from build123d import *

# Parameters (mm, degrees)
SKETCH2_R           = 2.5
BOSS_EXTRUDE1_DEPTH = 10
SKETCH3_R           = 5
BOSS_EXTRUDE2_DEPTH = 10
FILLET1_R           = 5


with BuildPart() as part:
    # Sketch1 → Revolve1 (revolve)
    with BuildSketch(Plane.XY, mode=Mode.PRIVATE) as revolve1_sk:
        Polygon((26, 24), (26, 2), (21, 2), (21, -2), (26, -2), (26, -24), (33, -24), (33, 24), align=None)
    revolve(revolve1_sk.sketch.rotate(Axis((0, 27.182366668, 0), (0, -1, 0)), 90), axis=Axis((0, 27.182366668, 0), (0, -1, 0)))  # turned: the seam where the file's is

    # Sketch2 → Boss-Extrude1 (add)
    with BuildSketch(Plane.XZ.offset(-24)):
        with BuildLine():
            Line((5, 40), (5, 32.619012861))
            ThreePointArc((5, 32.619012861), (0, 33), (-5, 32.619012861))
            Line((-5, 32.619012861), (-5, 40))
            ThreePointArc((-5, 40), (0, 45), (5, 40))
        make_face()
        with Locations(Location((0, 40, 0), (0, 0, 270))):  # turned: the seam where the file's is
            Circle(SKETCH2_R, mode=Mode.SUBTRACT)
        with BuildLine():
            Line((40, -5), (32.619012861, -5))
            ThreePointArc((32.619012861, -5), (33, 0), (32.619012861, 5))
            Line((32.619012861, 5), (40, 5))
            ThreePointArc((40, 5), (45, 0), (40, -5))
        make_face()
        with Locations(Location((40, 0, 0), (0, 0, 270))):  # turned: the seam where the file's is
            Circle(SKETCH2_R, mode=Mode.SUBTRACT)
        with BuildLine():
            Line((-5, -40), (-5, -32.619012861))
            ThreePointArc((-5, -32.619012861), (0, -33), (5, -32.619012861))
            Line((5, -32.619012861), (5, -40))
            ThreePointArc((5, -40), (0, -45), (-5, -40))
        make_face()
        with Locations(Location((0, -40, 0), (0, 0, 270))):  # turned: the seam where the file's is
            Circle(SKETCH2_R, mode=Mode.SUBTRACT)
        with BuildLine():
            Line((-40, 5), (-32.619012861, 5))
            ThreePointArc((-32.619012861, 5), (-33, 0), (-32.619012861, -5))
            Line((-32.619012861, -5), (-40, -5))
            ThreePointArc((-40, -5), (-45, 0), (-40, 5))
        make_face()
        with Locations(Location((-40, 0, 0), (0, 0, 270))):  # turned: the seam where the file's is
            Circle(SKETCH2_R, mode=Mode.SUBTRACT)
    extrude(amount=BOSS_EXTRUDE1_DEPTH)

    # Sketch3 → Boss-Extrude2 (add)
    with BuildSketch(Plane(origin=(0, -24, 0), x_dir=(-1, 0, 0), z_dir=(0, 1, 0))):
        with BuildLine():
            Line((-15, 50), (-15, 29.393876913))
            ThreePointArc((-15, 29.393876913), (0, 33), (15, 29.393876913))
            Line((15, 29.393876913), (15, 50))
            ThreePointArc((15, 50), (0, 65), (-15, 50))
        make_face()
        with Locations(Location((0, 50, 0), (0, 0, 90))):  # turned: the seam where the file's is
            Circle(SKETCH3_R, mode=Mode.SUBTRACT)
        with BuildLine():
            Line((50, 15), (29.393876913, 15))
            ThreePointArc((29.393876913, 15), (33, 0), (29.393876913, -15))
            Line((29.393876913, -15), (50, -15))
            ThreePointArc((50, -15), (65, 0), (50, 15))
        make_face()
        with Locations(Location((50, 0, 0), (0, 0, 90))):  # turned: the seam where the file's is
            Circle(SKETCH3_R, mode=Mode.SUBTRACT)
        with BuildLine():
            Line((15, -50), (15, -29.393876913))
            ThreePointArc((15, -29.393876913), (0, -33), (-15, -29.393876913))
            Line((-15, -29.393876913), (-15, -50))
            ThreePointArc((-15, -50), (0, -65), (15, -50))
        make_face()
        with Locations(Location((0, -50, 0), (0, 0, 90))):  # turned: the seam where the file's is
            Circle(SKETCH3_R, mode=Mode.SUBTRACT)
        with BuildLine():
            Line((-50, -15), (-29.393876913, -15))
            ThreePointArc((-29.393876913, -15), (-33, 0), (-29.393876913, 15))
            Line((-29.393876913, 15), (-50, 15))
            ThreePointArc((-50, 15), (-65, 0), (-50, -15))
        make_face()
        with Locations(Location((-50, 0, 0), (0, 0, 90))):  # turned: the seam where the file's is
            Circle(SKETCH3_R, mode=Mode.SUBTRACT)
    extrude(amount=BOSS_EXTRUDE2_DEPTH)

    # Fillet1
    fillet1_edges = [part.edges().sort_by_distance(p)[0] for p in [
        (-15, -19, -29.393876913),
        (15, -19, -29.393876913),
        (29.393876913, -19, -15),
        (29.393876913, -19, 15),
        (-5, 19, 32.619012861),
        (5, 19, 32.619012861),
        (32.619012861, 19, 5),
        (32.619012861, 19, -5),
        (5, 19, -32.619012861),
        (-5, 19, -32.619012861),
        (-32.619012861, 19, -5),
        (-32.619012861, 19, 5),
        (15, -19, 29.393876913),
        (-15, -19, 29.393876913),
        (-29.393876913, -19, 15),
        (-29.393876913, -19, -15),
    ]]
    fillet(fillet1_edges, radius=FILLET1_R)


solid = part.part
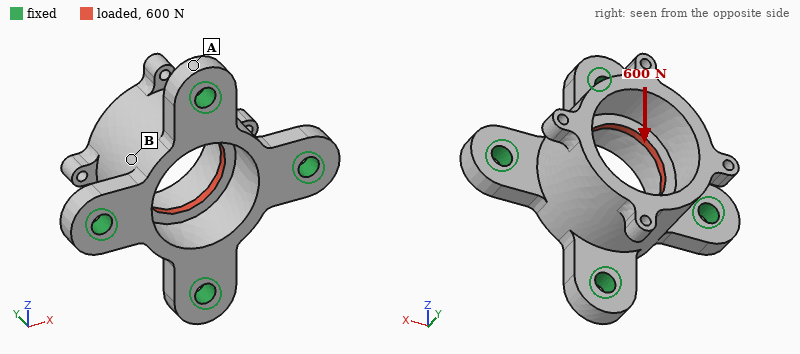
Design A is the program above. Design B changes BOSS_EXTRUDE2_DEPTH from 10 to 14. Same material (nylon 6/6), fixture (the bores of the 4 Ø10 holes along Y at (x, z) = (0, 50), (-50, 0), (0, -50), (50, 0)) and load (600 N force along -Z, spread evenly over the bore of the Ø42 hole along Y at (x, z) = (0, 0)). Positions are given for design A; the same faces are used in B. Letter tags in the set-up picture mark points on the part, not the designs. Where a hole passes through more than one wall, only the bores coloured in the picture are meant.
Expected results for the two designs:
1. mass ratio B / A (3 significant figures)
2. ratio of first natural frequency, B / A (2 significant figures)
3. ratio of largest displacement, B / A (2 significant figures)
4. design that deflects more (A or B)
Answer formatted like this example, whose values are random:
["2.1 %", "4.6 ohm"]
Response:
["1.13", "1.3", "0.58", "A"]
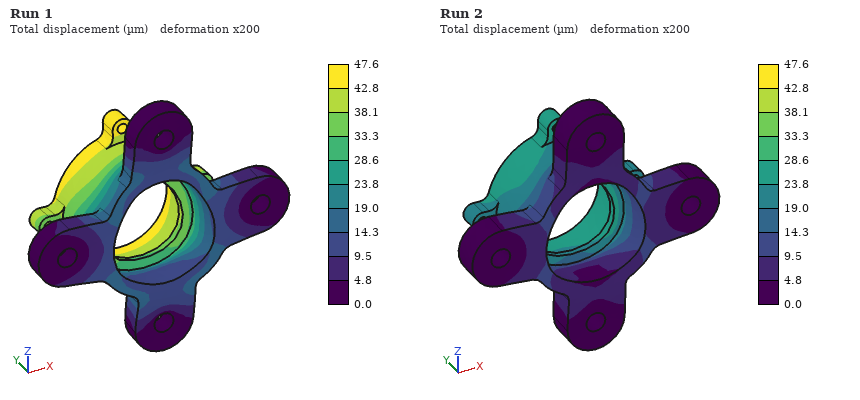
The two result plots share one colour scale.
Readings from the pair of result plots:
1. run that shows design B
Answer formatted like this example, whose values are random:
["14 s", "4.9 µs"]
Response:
["Run 2"]
